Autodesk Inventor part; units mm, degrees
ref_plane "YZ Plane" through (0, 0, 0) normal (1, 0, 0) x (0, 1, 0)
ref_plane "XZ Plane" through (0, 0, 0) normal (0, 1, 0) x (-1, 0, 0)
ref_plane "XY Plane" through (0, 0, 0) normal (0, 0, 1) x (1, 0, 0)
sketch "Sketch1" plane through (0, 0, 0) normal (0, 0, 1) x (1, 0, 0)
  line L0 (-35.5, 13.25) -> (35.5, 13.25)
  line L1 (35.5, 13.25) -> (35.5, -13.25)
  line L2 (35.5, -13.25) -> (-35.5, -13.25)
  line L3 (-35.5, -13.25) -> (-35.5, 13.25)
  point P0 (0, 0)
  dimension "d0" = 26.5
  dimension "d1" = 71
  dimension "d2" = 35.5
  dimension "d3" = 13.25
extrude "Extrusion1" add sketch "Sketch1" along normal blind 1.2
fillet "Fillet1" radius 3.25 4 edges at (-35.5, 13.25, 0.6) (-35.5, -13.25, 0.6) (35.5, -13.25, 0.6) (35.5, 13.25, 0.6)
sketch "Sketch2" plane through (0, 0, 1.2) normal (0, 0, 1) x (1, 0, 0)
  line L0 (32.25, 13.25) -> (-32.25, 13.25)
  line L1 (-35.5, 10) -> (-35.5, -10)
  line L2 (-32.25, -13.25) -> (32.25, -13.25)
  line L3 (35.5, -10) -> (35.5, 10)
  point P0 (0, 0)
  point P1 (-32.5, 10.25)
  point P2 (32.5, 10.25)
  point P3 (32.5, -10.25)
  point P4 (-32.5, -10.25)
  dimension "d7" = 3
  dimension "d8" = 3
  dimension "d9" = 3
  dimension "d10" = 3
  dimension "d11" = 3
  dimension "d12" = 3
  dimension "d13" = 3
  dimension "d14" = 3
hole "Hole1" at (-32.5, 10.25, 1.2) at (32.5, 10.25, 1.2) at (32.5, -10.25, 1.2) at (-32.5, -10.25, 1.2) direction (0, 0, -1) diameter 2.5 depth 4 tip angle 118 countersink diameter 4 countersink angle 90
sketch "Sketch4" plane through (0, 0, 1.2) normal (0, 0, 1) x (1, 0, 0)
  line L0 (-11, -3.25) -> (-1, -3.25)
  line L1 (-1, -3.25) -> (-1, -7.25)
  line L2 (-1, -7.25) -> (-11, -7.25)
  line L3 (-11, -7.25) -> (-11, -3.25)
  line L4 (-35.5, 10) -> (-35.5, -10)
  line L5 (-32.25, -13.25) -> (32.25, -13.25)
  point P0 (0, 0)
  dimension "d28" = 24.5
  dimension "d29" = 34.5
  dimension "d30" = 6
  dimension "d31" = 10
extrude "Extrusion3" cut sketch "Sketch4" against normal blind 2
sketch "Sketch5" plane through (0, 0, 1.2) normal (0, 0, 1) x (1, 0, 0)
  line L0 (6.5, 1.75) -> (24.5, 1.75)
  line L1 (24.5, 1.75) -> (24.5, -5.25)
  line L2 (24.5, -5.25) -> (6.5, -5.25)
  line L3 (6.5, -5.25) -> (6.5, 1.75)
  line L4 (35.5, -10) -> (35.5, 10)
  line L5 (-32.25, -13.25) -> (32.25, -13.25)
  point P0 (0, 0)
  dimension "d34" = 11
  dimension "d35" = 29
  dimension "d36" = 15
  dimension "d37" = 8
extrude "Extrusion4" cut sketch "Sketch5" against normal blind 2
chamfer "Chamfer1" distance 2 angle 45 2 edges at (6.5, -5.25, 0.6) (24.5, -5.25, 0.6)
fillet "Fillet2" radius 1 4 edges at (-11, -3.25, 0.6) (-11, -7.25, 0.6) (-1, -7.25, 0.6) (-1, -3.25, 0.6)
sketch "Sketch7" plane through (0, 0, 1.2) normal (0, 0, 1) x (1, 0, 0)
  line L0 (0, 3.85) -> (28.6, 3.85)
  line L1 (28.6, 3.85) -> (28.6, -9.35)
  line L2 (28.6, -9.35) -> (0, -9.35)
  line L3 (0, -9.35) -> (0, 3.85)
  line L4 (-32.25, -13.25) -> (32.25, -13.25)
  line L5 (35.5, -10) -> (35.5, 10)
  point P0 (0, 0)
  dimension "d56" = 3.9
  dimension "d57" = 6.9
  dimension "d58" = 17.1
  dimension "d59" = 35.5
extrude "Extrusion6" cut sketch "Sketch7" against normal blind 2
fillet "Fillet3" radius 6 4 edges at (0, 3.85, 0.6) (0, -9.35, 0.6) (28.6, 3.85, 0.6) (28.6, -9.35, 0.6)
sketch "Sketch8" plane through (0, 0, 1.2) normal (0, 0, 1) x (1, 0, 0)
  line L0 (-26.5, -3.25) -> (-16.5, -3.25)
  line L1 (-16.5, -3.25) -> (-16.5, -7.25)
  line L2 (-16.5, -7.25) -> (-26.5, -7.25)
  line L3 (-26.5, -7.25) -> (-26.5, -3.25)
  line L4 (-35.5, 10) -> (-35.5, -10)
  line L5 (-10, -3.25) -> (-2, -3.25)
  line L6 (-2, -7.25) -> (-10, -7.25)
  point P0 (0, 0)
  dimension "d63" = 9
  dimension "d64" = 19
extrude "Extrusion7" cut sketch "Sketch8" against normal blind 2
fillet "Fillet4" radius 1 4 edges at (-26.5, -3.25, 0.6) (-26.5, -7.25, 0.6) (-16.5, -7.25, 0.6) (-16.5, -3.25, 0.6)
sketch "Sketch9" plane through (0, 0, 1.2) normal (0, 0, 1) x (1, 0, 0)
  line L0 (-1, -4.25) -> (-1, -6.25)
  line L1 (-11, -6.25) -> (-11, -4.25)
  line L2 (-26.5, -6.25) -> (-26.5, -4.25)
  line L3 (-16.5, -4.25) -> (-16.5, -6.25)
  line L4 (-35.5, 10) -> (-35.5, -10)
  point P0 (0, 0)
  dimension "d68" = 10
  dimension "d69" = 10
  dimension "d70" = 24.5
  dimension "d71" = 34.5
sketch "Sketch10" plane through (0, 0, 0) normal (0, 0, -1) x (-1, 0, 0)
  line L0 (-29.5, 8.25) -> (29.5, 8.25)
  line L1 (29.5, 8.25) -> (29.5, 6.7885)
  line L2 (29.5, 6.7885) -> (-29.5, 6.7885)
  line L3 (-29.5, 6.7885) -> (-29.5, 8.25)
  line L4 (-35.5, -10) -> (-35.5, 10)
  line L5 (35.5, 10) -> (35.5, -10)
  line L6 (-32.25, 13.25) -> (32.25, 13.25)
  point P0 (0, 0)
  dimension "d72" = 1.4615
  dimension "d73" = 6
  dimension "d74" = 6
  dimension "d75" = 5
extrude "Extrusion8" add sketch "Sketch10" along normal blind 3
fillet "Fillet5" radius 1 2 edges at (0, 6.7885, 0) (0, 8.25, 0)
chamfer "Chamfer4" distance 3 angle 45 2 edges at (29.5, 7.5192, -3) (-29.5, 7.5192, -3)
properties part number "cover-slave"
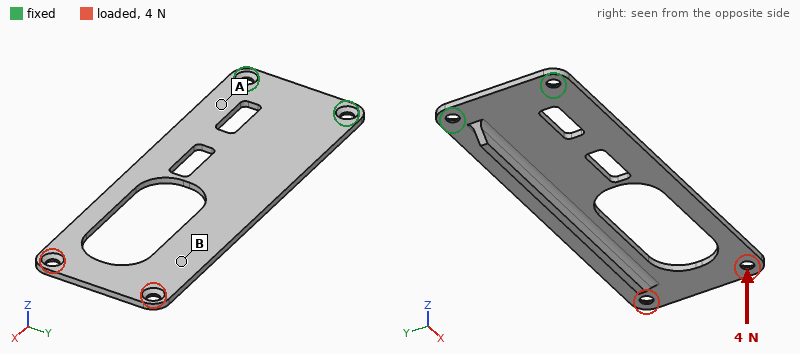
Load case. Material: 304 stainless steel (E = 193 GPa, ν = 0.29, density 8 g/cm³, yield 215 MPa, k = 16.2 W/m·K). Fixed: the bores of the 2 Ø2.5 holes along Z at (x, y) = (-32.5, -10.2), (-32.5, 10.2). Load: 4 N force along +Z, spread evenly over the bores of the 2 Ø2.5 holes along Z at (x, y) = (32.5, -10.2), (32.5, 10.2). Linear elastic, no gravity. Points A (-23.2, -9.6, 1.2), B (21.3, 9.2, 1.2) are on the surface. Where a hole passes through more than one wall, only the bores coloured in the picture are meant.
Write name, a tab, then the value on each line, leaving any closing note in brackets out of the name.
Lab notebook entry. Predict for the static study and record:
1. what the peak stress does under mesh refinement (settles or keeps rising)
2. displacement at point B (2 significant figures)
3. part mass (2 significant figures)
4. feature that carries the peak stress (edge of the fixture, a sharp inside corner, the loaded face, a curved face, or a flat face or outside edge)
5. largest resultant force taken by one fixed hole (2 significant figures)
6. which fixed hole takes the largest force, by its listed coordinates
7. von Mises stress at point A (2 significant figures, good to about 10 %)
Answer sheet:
what the peak stress does under mesh refinement	keeps rising
displacement at point B	0.22 mm
part mass	16 g
feature that carries the peak stress	edge of the fixture
largest resultant force taken by one fixed hole	3.3 N
which fixed hole takes the largest force, by its listed coordinates	(-32.5, -10.2)
von Mises stress at point A	23 MPa
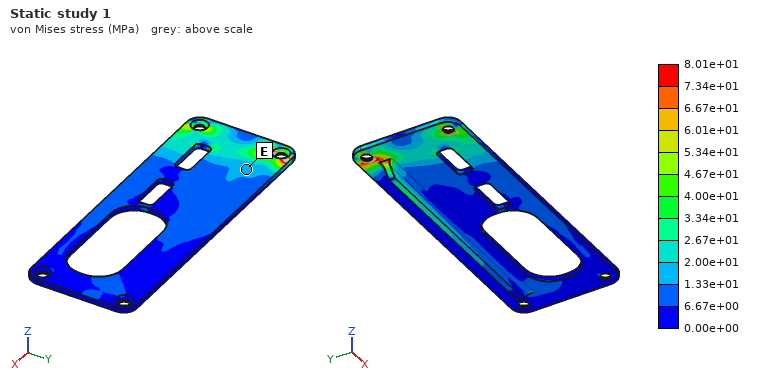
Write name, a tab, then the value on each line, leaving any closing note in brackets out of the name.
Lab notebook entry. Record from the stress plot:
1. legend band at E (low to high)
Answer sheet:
legend band at E	1.33e+01 to 2.00e+01 MPa
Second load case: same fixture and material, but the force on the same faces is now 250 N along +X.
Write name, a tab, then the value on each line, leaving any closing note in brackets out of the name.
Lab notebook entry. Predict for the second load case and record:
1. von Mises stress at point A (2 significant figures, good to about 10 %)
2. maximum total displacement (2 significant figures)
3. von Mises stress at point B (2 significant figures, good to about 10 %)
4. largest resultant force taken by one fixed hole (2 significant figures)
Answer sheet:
von Mises stress at point A	6.1 MPa
maximum total displacement	84 µm
von Mises stress at point B	9.4 MPa
largest resultant force taken by one fixed hole	130 N
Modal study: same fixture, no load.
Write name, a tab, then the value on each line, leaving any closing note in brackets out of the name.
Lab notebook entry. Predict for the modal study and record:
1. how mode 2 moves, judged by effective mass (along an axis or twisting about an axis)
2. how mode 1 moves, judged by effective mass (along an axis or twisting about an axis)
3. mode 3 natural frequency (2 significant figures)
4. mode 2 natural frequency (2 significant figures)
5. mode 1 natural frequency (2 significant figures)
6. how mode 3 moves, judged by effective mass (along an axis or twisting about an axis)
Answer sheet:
how mode 2 moves, judged by effective mass	twisting about X
how mode 1 moves, judged by effective mass	along Z
mode 3 natural frequency	2100 Hz
mode 2 natural frequency	1200 Hz
mode 1 natural frequency	290 Hz
how mode 3 moves, judged by effective mass	along Z
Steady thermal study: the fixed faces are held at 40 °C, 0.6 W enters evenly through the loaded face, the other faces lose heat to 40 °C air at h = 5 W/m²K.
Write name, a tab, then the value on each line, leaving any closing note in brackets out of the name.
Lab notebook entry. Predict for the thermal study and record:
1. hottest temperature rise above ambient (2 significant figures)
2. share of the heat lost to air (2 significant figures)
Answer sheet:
hottest temperature rise above ambient	67 K
share of the heat lost to air	63 %
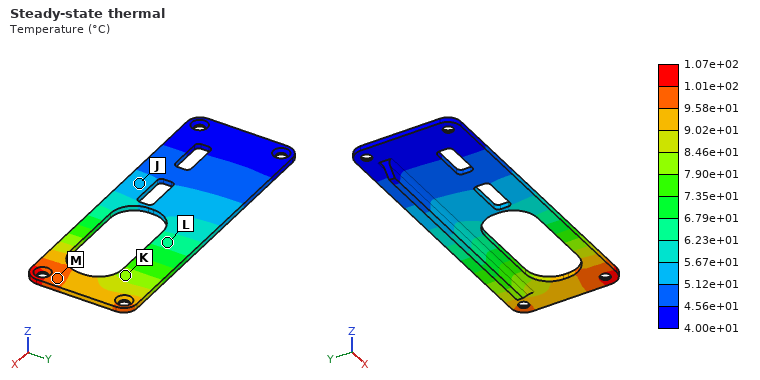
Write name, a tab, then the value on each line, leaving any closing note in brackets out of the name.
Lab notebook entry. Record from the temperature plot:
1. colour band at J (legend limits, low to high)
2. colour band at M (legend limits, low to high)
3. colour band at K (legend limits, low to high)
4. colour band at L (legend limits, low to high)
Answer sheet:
colour band at J	5.12e+01 to 5.67e+01 °C
colour band at M	9.58e+01 to 1.01e+02 °C
colour band at K	7.90e+01 to 8.46e+01 °C
colour band at L	6.23e+01 to 6.79e+01 °C
